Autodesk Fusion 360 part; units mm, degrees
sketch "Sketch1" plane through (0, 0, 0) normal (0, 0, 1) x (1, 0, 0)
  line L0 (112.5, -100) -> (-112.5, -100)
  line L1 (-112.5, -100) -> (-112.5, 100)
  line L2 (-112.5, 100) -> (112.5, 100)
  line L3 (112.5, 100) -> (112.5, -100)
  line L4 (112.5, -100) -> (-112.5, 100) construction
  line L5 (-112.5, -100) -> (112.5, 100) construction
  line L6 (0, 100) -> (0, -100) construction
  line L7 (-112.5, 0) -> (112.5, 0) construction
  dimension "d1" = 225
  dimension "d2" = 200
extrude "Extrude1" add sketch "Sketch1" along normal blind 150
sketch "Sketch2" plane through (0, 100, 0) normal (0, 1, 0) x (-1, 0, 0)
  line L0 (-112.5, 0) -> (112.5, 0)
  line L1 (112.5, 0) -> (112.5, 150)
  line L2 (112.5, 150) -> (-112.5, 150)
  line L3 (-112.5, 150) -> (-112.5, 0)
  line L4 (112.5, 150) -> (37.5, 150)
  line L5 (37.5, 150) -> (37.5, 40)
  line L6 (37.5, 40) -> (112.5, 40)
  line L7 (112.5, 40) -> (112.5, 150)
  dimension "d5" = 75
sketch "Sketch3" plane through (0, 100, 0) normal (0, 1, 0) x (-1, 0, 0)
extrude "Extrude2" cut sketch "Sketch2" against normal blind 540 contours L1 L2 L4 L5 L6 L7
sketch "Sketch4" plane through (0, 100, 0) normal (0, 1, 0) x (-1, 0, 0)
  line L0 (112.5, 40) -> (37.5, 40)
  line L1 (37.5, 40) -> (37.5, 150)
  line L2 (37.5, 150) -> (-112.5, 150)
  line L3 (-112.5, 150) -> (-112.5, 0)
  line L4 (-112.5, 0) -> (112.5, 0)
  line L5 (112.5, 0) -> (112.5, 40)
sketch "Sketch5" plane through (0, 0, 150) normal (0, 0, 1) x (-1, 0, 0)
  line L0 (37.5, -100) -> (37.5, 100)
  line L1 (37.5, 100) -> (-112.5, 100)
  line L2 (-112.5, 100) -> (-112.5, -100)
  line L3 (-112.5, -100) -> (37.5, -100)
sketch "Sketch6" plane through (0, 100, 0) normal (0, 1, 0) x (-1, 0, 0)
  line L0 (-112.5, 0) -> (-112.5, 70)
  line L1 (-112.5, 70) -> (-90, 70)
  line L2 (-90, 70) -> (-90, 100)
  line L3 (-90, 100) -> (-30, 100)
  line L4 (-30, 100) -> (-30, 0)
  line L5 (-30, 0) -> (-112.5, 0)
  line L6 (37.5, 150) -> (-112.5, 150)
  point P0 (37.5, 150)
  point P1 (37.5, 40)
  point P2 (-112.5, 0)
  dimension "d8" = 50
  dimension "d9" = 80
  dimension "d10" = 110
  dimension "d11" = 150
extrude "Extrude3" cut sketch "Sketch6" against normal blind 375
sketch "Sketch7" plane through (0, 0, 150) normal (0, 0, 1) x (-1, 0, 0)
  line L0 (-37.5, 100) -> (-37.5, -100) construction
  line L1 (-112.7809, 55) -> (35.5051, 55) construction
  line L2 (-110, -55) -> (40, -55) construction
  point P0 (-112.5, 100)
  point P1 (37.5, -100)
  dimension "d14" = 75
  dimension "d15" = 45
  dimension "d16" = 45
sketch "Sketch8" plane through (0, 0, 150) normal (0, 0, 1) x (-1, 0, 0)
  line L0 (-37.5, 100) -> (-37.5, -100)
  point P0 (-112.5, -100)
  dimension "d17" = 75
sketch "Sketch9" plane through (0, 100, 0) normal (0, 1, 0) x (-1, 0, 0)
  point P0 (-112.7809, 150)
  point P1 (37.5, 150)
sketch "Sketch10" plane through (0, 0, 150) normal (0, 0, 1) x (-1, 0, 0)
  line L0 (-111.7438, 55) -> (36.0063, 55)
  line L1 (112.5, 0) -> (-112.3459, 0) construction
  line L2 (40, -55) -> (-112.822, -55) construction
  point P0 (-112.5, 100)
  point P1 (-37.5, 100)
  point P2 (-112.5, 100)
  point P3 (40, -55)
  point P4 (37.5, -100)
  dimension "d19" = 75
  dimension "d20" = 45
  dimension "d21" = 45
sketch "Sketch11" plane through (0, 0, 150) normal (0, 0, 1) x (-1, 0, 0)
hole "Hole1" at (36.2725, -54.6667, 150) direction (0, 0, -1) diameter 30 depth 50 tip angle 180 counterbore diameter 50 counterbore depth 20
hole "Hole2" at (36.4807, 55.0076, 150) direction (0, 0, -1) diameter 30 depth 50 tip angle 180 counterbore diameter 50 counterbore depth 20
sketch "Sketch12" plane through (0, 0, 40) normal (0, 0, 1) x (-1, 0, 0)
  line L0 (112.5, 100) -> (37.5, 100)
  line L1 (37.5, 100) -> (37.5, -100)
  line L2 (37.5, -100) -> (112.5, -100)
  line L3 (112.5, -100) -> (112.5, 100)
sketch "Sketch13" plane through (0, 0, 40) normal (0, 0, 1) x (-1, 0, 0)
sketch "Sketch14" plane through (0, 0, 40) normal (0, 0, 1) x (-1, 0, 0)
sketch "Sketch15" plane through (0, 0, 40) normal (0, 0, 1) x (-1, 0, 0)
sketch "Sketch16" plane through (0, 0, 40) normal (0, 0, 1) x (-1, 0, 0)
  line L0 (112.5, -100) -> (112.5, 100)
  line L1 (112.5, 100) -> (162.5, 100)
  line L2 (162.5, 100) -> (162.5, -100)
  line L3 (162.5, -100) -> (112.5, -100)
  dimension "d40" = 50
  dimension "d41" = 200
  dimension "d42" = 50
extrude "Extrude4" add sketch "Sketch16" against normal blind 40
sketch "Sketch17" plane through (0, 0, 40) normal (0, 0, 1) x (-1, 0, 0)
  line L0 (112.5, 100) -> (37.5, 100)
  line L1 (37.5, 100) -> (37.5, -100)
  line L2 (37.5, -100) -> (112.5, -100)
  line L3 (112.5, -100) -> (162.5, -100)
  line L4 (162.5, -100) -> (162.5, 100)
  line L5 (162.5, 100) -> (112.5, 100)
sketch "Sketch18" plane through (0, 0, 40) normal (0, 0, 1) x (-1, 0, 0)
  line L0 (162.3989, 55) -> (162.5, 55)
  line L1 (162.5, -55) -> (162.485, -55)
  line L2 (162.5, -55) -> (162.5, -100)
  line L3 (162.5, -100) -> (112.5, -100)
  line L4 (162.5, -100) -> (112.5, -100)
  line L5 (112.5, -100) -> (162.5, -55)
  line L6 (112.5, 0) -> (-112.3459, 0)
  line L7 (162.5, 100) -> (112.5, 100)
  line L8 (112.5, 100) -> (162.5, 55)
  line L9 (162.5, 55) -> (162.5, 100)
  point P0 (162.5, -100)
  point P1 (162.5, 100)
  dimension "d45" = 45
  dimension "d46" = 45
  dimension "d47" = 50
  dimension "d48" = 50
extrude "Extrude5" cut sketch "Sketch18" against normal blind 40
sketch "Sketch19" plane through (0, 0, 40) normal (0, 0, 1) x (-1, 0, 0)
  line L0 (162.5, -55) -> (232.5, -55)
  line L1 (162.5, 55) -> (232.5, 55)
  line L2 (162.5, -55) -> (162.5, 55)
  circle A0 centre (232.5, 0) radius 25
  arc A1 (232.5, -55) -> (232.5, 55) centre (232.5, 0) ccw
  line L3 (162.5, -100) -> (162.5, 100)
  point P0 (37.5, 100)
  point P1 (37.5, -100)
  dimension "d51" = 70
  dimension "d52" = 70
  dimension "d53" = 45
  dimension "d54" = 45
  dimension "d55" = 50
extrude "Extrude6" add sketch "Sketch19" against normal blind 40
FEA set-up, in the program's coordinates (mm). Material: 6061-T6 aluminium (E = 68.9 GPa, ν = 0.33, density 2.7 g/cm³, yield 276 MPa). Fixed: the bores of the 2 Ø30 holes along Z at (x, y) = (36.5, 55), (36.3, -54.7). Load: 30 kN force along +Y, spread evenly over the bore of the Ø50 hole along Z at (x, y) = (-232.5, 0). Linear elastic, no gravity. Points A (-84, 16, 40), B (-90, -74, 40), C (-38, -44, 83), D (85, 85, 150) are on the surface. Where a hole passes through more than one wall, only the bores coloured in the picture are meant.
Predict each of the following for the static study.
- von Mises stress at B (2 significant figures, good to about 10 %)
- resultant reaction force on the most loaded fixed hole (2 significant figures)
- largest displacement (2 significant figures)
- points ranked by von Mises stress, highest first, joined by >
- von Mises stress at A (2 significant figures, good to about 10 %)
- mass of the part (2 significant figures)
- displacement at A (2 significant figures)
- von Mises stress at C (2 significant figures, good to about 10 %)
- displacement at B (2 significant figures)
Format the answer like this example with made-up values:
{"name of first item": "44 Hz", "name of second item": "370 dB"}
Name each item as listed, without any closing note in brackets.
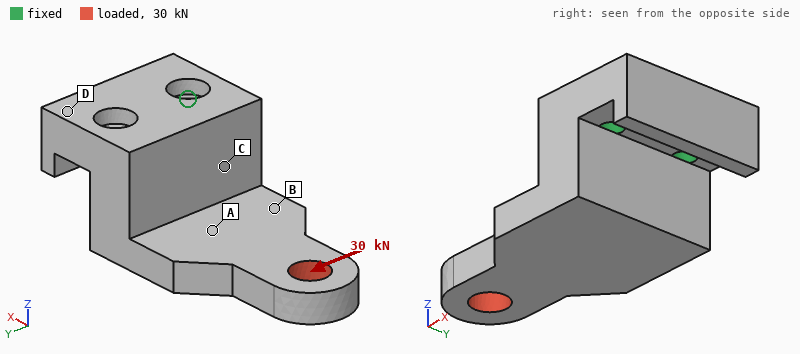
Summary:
{"von Mises stress at B": "23 MPa", "resultant reaction force on the most loaded fixed hole": "71 kN", "largest displacement": "0.54 mm", "points ranked by von Mises stress, highest first, joined by >": "C > B > A > D", "von Mises stress at A": "13 MPa", "mass of the part": "11 kg", "displacement at A": "0.13 mm", "von Mises stress at C": "32 MPa", "displacement at B": "0.18 mm"}
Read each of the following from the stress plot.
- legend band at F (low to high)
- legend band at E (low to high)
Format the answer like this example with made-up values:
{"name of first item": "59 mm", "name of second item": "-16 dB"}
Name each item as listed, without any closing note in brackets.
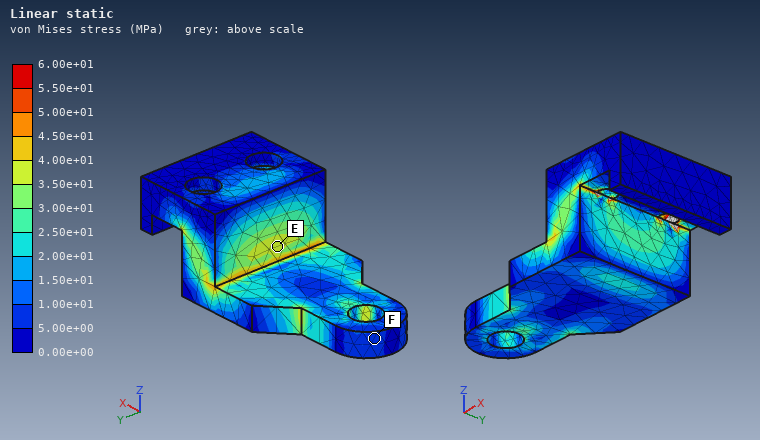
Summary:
{"legend band at F": "5.00e+00 to 1.00e+01 MPa", "legend band at E": "3.50e+01 to 4.00e+01 MPa"}
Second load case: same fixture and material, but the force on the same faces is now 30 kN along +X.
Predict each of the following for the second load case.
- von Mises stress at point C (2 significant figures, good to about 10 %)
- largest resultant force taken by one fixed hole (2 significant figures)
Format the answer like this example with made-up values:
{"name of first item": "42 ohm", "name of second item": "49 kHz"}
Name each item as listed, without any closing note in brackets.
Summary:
{"von Mises stress at point C": "12 MPa", "largest resultant force taken by one fixed hole": "15 kN"}
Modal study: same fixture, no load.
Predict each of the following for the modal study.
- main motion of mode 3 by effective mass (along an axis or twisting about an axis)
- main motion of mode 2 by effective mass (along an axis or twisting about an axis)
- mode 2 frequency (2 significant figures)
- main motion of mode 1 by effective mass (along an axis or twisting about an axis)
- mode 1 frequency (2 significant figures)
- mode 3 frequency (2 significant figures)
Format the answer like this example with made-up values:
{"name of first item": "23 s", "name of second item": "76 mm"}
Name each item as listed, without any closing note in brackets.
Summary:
{"main motion of mode 3 by effective mass": "along X", "main motion of mode 2 by effective mass": "along Y", "mode 2 frequency": "1100 Hz", "main motion of mode 1 by effective mass": "along Z", "mode 1 frequency": "440 Hz", "mode 3 frequency": "1200 Hz"}
